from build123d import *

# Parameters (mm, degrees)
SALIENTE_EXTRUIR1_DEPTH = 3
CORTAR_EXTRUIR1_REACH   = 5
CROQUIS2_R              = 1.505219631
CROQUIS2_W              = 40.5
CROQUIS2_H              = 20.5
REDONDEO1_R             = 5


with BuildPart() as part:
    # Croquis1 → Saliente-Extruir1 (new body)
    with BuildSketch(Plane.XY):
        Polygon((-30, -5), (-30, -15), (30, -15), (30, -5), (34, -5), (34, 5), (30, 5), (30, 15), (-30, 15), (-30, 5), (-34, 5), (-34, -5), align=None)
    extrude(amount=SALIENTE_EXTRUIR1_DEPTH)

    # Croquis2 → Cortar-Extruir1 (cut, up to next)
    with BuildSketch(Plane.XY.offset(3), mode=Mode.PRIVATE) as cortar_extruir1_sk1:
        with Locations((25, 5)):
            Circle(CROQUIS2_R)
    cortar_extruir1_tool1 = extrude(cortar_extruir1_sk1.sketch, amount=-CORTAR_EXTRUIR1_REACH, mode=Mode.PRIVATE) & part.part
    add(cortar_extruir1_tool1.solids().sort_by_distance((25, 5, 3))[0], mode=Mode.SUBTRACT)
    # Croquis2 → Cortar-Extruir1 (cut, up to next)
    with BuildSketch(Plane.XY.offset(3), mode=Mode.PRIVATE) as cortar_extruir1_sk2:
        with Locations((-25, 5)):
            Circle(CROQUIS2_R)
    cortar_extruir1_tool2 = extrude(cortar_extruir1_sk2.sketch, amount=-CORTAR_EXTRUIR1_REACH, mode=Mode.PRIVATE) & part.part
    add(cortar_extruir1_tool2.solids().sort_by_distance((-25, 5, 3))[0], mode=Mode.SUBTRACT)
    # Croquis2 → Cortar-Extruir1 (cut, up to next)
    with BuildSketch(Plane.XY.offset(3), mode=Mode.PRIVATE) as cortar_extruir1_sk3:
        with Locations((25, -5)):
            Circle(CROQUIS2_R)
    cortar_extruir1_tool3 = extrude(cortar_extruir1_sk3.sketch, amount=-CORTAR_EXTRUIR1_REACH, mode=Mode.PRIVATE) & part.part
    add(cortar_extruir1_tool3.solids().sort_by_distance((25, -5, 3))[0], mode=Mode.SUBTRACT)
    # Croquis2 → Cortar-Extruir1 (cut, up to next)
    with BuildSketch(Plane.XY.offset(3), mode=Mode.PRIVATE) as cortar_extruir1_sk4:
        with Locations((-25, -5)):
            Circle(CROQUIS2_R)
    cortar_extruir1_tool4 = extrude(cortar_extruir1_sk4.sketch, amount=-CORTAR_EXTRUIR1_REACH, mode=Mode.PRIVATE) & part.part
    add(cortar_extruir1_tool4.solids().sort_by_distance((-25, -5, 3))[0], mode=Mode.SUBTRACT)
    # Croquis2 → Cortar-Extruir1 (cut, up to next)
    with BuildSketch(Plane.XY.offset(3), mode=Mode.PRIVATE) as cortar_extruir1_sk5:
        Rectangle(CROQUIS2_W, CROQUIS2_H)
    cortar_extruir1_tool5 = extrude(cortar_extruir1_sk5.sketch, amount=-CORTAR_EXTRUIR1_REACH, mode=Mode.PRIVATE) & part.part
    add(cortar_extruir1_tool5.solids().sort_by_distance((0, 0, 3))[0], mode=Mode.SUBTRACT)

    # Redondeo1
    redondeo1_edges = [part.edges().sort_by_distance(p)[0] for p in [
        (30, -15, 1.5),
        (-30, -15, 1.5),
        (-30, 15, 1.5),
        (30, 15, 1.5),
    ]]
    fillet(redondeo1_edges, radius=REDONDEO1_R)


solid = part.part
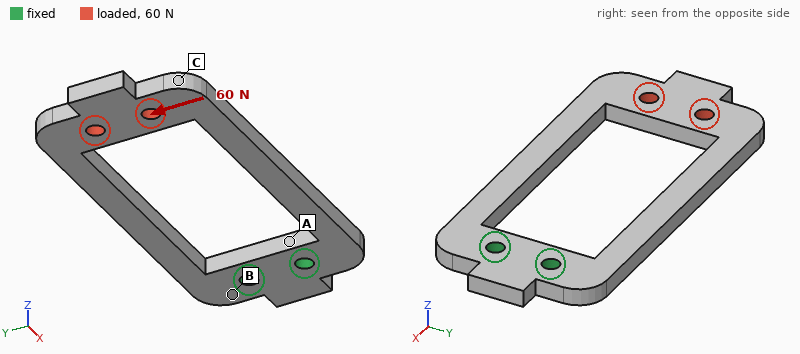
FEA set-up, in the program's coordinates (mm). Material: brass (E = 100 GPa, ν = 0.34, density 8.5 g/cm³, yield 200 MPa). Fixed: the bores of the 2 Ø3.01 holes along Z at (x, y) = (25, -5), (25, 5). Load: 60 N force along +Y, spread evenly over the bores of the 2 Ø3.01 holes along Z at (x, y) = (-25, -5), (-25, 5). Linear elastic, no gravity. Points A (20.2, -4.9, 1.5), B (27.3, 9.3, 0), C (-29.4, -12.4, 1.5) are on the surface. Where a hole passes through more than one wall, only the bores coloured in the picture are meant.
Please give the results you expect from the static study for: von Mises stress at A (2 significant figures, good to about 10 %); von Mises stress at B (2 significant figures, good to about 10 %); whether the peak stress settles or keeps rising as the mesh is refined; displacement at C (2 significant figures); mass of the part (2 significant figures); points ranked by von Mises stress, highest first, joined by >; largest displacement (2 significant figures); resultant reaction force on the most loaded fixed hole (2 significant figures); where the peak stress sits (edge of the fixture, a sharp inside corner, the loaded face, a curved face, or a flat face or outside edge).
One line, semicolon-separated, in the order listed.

18 MPa; 13 MPa; keeps rising; 0.12 mm; 25 g; A > B > C; 0.12 mm; 180 N; a sharp inside corner
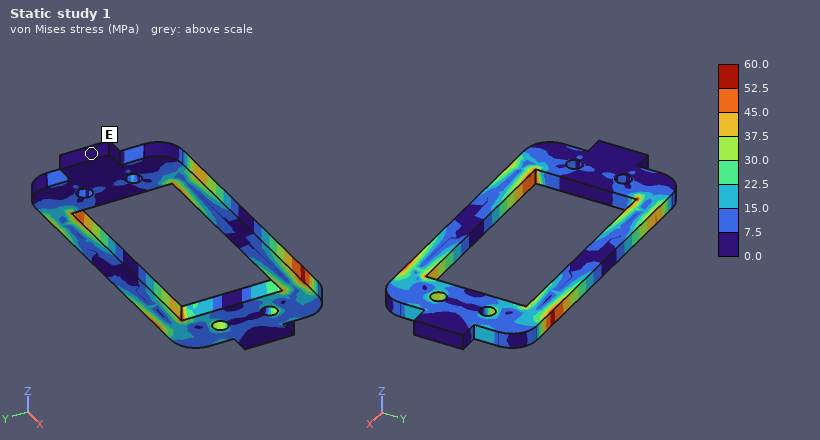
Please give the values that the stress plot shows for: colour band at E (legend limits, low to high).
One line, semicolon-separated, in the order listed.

0.0 to 7.5 MPa
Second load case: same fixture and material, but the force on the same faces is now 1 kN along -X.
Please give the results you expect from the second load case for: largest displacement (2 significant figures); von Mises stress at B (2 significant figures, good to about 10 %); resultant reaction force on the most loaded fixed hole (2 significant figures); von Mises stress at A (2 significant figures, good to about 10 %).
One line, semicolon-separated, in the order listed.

38 µm; 37 MPa; 500 N; 58 MPa
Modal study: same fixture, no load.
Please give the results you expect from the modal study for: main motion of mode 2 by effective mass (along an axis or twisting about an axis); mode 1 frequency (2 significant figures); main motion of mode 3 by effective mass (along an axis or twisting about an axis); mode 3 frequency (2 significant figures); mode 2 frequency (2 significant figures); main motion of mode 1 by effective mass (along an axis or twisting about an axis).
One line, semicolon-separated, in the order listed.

along Y; 350 Hz; twisting about X; 1200 Hz; 1100 Hz; along Z
